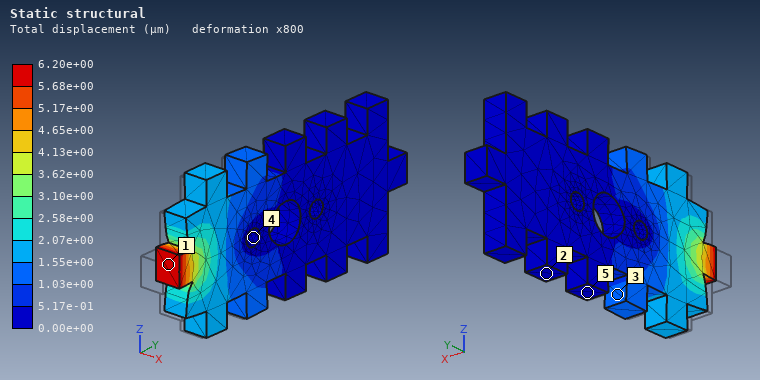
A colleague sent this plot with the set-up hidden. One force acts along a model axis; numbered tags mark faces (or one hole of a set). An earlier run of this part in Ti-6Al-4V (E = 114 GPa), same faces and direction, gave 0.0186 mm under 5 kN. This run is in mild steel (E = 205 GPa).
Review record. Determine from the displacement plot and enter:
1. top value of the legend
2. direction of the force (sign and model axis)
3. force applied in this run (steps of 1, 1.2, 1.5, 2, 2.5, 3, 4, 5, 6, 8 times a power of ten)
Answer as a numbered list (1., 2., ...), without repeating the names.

1. 6.20e+00 µm
2. +Y
3. 3 kN
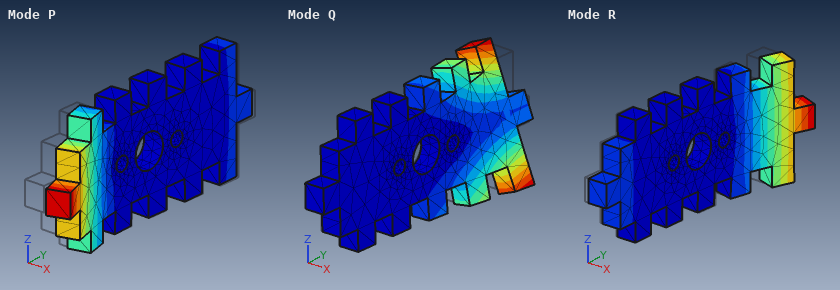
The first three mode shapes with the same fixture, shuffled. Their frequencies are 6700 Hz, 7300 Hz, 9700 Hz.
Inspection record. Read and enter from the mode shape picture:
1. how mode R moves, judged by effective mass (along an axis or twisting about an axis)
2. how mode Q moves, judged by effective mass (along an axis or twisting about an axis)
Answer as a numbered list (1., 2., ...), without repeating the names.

1. along X
2. twisting about Y
